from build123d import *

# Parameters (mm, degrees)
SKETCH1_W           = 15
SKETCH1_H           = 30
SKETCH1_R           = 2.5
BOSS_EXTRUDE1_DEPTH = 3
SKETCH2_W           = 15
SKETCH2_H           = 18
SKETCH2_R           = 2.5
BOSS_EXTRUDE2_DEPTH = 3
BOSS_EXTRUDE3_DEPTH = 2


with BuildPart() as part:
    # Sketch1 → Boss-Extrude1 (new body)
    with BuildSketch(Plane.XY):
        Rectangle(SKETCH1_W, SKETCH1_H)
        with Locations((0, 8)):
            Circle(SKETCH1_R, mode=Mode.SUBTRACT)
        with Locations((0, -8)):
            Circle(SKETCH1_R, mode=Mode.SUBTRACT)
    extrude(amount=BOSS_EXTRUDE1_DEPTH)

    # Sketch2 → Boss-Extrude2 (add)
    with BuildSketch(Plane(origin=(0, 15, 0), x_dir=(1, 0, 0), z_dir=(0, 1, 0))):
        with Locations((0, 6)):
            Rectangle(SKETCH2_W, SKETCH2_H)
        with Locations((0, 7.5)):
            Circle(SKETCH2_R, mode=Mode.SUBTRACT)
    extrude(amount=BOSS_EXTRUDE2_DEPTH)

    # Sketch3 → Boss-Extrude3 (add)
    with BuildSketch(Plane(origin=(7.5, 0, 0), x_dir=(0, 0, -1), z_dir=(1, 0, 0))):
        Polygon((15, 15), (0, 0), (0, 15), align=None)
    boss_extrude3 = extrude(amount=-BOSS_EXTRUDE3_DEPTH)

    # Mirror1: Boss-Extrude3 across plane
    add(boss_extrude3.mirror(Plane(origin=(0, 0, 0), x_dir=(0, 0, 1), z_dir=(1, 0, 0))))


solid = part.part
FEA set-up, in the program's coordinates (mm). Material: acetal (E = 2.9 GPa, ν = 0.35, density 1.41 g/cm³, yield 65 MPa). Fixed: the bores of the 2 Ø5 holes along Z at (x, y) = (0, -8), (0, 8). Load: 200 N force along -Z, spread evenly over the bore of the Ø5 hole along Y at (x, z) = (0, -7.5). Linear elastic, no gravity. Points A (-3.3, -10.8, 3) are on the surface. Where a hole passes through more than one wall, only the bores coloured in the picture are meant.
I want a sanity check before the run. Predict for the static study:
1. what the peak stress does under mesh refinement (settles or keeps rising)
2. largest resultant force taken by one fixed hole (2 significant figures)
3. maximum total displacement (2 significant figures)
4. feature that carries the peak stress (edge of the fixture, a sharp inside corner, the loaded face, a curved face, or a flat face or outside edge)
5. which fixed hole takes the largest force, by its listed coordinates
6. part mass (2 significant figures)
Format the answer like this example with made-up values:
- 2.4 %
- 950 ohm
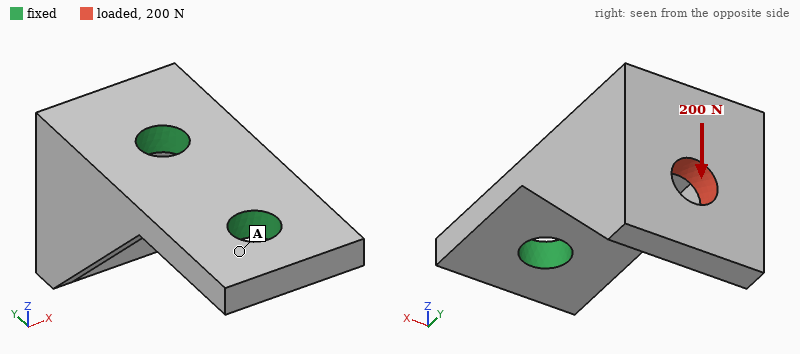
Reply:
- keeps rising
- 240 N
- 0.30 mm
- edge of the fixture
- (0, 8)
- 3.4 g
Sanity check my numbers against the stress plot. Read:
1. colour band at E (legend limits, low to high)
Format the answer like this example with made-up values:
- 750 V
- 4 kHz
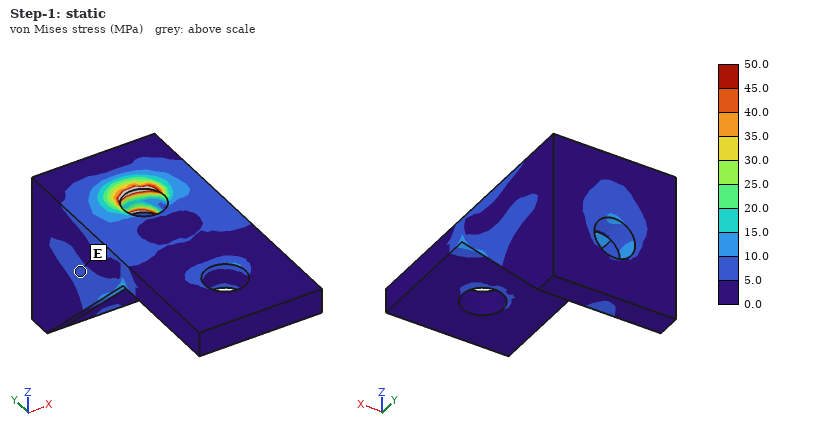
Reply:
- 5.0 to 10.0 MPa
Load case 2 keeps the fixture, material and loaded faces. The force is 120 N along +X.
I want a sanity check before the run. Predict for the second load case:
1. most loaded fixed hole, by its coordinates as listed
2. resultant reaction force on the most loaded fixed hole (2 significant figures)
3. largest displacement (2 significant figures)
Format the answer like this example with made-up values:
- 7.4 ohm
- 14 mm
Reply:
- (0, 8)
- 150 N
- 0.45 mm
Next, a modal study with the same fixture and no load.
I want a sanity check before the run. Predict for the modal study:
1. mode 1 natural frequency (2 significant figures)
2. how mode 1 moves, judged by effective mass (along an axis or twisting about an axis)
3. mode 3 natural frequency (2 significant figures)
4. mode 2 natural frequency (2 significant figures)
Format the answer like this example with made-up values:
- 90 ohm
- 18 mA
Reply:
- 2600 Hz
- along X
- 7400 Hz
- 3500 Hz
